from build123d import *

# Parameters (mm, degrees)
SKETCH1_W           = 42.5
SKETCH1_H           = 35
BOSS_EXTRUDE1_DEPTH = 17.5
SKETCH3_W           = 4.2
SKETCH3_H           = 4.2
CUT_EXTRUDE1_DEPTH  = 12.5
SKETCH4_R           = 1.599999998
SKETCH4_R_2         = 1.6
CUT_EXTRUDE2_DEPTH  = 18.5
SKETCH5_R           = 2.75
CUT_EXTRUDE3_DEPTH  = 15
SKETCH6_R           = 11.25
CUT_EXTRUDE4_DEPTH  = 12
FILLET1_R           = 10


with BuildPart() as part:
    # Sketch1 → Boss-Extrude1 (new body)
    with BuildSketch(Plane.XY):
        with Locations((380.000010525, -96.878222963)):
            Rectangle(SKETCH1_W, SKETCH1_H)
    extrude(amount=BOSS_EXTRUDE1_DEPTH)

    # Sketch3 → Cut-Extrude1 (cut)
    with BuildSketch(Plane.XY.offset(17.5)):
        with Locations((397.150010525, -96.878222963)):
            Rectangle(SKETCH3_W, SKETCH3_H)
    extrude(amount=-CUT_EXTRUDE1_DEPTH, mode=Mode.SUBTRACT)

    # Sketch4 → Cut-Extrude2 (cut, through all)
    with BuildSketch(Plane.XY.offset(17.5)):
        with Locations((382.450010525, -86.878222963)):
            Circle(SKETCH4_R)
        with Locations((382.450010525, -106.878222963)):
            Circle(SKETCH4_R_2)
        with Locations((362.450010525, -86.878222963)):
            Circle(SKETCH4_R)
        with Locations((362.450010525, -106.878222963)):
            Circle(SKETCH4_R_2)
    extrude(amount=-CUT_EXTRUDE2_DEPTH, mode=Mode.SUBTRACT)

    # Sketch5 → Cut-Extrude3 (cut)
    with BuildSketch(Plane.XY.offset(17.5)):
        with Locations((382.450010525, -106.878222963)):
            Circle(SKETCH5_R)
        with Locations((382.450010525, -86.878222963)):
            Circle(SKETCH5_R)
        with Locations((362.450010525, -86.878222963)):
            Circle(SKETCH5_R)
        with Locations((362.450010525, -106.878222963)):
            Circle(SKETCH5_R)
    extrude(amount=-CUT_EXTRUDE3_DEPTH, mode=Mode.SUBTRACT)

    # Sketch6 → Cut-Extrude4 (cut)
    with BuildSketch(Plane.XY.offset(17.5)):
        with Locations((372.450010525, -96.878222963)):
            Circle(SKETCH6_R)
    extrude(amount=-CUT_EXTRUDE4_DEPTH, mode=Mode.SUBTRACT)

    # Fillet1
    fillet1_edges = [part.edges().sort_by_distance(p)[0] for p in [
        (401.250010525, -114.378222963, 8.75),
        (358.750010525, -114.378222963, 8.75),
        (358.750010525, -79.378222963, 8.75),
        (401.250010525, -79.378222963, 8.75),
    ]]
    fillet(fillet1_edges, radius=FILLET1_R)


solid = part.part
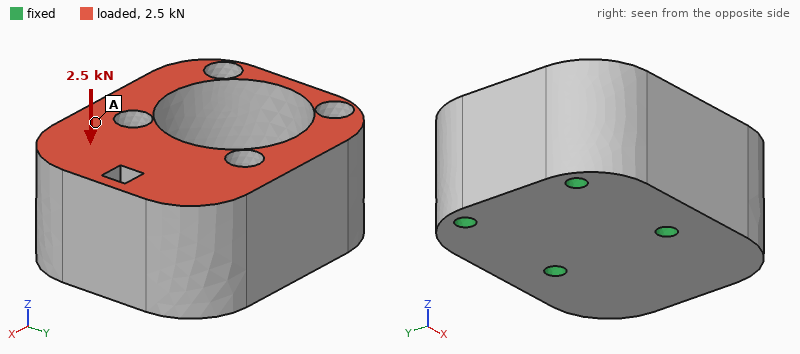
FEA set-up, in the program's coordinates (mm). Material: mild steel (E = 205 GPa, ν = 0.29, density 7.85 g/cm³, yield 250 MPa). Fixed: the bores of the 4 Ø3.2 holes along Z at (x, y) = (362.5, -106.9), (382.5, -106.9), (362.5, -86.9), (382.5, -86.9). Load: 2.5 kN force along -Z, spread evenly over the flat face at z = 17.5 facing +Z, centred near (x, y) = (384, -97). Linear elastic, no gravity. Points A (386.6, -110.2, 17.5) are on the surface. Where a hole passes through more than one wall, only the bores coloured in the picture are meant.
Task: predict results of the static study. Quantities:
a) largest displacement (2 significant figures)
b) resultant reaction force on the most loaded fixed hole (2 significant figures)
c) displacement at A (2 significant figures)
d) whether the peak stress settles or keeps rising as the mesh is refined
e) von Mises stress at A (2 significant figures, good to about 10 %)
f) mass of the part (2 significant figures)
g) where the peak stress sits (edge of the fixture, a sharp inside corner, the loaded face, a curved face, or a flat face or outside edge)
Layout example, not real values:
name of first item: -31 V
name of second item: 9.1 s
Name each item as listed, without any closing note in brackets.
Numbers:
largest displacement: 6.4 µm
resultant reaction force on the most loaded fixed hole: 1.3 kN
displacement at A: 3.7 µm
whether the peak stress settles or keeps rising as the mesh is refined: keeps rising
von Mises stress at A: 13 MPa
mass of the part: 140 g
where the peak stress sits: edge of the fixture
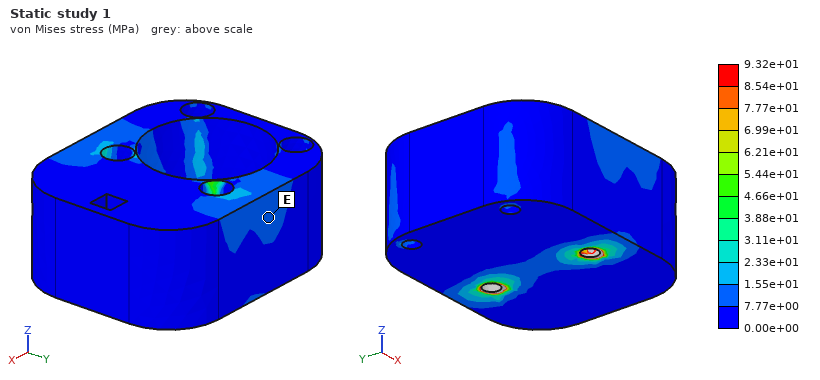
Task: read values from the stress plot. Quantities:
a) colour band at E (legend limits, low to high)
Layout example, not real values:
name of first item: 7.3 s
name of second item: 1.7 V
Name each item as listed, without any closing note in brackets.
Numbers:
colour band at E: 7.77e+00 to 1.55e+01 MPa
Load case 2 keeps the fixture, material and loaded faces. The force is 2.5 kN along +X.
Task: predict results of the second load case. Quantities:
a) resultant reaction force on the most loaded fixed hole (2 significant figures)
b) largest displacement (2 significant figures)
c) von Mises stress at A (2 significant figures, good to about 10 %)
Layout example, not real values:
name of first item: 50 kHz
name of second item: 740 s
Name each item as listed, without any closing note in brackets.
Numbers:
resultant reaction force on the most loaded fixed hole: 1.2 kN
largest displacement: 11 µm
von Mises stress at A: 29 MPa
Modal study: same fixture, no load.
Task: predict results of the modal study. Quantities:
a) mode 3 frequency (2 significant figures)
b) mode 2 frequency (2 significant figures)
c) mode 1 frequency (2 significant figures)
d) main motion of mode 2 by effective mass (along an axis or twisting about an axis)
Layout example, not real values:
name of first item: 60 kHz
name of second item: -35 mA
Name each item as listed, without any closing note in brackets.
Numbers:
mode 3 frequency: 19 kHz
mode 2 frequency: 13 kHz
mode 1 frequency: 9900 Hz
main motion of mode 2 by effective mass: along Y
